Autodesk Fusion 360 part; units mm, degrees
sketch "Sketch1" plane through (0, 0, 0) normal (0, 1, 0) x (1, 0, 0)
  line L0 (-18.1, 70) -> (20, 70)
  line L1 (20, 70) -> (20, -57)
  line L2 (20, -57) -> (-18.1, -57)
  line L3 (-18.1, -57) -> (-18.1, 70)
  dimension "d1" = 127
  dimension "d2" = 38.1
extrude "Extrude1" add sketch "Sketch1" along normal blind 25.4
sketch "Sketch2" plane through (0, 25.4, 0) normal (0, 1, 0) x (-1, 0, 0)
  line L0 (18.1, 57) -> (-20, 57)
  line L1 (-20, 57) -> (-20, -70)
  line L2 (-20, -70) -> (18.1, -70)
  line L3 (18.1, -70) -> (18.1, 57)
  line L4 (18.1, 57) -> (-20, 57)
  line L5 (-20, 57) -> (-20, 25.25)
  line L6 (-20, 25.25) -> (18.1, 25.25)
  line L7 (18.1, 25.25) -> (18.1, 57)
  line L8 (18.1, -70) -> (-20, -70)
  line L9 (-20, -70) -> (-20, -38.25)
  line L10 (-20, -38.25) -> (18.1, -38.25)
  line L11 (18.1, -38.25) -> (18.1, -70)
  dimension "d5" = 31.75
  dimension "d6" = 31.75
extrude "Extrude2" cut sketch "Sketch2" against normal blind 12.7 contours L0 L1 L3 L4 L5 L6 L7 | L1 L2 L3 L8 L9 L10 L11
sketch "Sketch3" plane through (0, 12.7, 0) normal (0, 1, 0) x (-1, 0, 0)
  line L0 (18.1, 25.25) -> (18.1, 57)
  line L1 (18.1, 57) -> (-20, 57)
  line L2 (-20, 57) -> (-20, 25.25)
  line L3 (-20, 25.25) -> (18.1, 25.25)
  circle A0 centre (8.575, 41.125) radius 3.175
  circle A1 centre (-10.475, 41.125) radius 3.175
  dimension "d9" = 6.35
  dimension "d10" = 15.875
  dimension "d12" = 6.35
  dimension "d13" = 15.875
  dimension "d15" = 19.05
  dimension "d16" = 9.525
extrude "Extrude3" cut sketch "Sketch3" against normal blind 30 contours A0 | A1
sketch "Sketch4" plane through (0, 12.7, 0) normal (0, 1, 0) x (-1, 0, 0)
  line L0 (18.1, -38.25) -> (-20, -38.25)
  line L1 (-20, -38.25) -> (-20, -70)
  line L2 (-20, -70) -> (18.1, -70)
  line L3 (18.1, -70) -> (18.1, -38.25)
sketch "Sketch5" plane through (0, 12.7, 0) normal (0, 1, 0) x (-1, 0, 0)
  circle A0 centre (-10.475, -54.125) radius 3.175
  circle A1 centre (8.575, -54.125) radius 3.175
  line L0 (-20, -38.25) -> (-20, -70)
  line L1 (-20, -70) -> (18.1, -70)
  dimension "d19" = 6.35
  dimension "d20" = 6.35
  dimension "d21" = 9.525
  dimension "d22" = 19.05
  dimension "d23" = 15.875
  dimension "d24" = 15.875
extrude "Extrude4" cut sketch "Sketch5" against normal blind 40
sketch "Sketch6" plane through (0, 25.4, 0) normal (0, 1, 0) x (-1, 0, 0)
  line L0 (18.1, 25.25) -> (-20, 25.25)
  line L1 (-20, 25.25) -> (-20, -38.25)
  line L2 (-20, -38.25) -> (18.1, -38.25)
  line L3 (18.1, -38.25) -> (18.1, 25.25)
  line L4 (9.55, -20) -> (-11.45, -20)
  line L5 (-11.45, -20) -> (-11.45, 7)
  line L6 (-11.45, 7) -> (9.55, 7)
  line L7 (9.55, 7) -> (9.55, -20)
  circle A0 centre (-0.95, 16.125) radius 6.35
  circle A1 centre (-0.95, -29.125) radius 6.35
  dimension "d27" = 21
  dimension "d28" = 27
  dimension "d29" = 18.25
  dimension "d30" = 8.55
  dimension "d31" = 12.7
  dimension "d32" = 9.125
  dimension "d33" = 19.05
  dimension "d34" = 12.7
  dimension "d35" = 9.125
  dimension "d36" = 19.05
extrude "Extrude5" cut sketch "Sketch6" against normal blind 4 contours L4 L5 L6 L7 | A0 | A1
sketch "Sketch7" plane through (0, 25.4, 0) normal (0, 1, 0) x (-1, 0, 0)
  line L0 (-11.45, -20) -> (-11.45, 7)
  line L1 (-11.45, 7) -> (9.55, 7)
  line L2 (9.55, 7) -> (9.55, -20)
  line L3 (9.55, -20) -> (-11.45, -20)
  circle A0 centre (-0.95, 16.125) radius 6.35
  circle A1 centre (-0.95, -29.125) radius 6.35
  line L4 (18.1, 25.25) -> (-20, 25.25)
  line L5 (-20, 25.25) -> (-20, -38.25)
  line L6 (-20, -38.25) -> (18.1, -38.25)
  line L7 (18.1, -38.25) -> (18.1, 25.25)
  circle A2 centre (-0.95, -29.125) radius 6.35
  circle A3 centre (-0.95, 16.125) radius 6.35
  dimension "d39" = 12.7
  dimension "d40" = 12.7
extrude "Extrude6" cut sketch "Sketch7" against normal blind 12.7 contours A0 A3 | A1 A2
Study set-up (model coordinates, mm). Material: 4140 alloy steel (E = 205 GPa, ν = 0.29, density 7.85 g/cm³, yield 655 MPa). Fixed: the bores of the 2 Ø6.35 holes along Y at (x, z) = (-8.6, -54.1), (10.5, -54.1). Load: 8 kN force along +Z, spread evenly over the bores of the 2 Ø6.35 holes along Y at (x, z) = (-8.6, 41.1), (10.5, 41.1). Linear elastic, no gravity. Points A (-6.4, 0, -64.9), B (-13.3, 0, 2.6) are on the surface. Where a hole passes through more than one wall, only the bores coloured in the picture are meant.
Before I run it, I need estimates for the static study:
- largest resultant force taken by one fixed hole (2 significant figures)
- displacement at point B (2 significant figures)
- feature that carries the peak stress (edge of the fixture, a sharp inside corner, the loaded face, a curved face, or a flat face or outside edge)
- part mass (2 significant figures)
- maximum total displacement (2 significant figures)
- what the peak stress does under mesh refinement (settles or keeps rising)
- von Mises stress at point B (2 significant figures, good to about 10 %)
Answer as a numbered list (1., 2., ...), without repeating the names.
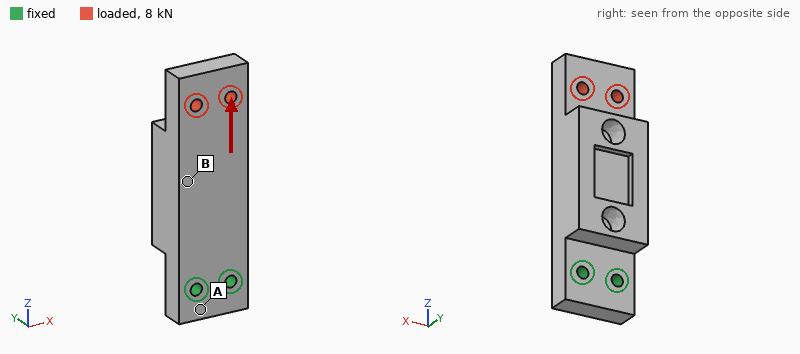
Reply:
1. 4.0 kN
2. 6.5 µm
3. edge of the fixture
4. 670 g
5. 20 µm
6. keeps rising
7. 21 MPa
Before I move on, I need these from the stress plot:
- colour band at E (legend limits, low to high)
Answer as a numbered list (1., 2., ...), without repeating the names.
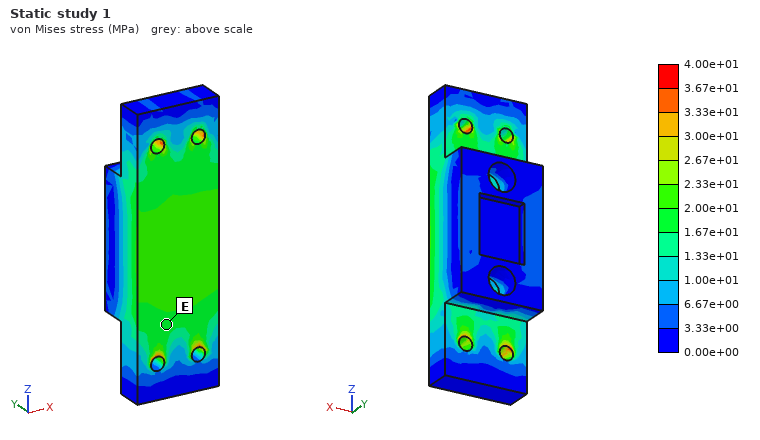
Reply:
1. 1.67e+01 to 2.00e+01 MPa
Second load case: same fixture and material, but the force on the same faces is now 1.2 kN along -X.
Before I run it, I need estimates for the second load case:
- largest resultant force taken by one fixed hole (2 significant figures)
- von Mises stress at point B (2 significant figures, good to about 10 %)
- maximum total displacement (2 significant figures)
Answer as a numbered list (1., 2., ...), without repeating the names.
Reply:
1. 5.0 kN
2. 8.2 MPa
3. 37 µm
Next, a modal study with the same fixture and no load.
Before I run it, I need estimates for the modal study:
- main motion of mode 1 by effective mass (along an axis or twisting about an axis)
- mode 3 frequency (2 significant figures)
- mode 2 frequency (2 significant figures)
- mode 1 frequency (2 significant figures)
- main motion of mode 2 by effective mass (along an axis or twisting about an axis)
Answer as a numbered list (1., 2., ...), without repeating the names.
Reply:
1. along Y
2. 4700 Hz
3. 2200 Hz
4. 950 Hz
5. along X
